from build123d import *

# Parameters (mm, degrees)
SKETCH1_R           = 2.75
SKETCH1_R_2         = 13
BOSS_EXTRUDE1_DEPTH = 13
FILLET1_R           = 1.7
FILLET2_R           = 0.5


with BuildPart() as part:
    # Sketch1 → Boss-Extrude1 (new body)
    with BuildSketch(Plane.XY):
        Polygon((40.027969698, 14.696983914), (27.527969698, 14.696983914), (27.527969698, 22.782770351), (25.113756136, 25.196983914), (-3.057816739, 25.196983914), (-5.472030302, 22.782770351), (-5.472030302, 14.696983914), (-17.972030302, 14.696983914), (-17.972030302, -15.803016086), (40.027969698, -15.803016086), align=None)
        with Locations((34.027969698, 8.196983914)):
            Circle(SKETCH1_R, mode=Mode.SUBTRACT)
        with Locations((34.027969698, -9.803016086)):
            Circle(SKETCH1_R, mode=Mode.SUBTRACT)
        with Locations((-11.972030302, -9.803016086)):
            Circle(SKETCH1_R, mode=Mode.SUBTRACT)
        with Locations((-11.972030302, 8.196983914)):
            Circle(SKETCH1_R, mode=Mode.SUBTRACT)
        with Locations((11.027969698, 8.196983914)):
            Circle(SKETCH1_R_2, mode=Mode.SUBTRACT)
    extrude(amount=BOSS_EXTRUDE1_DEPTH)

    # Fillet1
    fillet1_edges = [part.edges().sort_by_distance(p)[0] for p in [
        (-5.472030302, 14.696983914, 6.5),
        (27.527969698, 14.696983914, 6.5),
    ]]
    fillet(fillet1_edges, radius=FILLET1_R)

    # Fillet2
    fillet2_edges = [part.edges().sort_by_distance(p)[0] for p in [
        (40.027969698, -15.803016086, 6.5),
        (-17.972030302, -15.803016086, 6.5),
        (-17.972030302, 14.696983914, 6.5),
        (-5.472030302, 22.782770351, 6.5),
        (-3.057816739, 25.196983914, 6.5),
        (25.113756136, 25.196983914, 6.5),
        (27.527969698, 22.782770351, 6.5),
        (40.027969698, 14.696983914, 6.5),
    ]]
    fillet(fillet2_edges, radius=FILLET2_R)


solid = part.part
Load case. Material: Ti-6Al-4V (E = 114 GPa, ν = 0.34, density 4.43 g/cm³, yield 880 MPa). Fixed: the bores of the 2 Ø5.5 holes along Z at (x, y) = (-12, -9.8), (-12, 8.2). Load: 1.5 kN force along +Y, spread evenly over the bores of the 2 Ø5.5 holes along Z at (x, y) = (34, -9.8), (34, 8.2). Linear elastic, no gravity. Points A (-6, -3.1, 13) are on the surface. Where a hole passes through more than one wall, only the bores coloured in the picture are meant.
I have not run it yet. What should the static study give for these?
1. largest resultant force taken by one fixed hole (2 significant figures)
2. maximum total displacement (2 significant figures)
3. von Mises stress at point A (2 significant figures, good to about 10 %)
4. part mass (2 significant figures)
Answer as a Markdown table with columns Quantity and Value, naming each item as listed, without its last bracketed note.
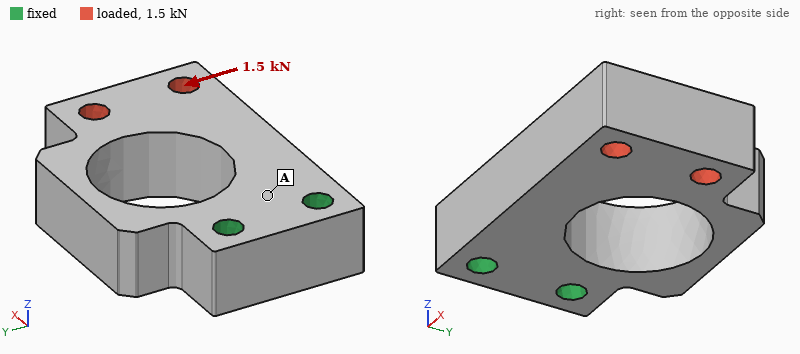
| Quantity | Value |
|---|---|
| largest resultant force taken by one fixed hole | 3.2 kN |
| maximum total displacement | 68 µm |
| von Mises stress at point A | 18 MPa |
| part mass | 86 g |
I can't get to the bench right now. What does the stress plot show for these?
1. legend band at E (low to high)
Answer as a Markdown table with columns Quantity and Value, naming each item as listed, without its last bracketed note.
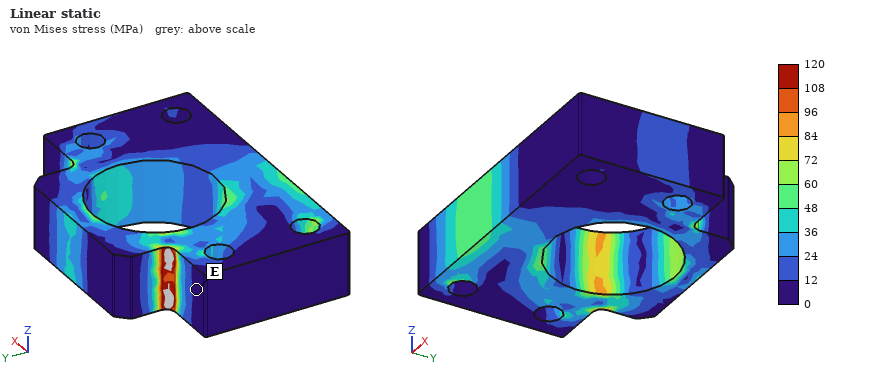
| Quantity | Value |
|---|---|
| legend band at E | 0 to 12 MPa |
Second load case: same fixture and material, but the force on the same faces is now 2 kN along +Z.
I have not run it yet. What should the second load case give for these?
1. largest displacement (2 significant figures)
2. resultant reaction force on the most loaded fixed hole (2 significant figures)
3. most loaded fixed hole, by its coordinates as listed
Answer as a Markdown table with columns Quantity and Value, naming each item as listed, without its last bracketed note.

| Quantity | Value |
|---|---|
| largest displacement | 0.22 mm |
| resultant reaction force on the most loaded fixed hole | 1.2 kN |
| most loaded fixed hole, by its coordinates as listed | (-12, -9.8) |
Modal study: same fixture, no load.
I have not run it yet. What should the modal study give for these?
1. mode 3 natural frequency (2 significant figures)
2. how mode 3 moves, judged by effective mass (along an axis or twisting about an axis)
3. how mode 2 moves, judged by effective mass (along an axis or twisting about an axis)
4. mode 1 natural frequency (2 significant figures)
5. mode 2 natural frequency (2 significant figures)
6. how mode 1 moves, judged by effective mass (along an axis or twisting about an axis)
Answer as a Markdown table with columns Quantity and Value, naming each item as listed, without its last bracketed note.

| Quantity | Value |
|---|---|
| mode 3 natural frequency | 7500 Hz |
| how mode 3 moves, judged by effective mass | twisting about X |
| how mode 2 moves, judged by effective mass | along Y |
| mode 1 natural frequency | 3100 Hz |
| mode 2 natural frequency | 4400 Hz |
| how mode 1 moves, judged by effective mass | along Z |
